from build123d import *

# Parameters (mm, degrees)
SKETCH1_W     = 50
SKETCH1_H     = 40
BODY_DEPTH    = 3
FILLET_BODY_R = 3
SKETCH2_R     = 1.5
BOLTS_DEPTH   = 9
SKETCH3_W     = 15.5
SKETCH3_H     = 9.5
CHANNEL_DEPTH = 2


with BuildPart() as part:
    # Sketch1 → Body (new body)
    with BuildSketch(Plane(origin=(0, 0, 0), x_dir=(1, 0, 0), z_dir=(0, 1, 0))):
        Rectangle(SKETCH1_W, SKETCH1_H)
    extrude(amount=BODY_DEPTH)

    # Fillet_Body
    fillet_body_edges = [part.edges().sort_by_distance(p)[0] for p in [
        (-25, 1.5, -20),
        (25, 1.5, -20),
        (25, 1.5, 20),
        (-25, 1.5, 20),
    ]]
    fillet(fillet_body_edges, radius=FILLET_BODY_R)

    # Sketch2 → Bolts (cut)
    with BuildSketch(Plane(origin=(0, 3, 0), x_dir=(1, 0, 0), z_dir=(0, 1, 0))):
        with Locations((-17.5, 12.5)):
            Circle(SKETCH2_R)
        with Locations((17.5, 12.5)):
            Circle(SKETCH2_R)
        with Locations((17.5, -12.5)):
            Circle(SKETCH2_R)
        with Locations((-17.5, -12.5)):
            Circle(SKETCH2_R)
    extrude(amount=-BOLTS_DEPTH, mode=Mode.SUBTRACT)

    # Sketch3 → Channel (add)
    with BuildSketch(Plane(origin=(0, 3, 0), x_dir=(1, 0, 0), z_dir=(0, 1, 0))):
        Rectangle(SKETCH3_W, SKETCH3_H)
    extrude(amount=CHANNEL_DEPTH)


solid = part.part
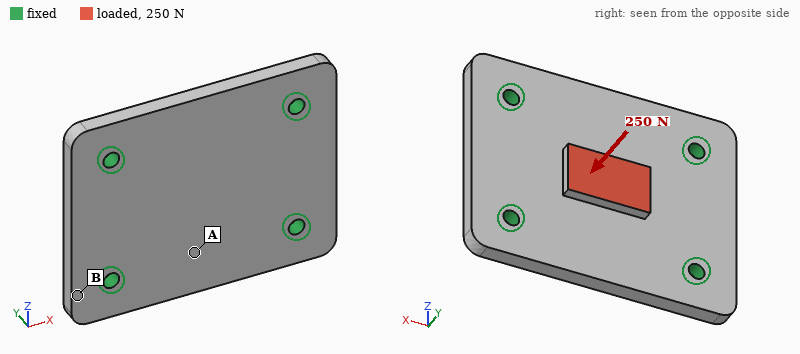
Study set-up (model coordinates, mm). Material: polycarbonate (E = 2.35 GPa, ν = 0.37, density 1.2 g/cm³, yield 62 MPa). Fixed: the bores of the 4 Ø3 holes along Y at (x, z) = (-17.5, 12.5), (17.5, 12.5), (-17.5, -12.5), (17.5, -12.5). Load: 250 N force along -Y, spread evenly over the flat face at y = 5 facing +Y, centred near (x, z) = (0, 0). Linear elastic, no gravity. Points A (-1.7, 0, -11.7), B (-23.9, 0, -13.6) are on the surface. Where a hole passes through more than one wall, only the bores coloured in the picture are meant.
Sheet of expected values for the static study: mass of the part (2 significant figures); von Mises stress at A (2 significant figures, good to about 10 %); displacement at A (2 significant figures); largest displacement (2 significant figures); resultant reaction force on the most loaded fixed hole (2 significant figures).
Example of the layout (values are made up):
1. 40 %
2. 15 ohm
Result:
1. 7.4 g
2. 7.5 MPa
3. 0.20 mm
4. 0.29 mm
5. 65 N
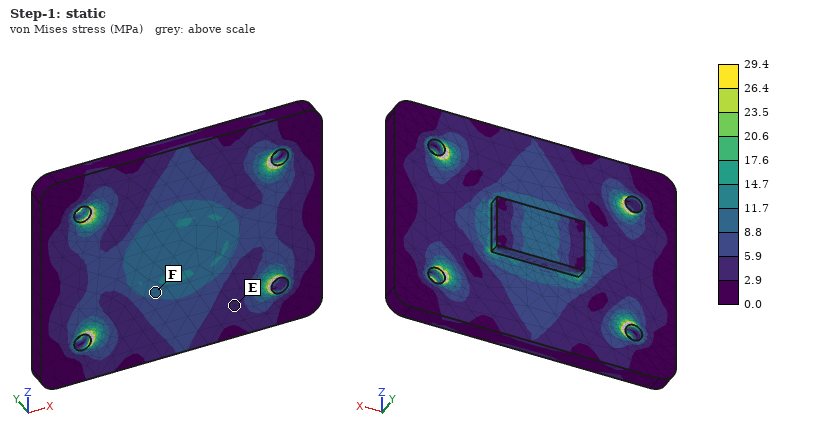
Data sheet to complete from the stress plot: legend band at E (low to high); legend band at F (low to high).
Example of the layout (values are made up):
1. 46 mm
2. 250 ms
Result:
1. 2.9 to 5.9 MPa
2. 8.8 to 11.7 MPa
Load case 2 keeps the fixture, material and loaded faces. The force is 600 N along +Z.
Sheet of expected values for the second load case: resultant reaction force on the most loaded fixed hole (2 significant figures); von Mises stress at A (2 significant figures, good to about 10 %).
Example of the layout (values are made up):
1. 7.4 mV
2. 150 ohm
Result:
1. 180 N
2. 7.1 MPa
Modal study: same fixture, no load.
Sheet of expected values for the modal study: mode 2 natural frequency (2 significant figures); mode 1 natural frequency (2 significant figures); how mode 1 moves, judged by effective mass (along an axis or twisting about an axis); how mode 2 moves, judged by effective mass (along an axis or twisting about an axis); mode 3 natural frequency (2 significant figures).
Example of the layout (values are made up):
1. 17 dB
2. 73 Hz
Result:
1. 3800 Hz
2. 3100 Hz
3. along Y
4. twisting about X
5. 4900 Hz
